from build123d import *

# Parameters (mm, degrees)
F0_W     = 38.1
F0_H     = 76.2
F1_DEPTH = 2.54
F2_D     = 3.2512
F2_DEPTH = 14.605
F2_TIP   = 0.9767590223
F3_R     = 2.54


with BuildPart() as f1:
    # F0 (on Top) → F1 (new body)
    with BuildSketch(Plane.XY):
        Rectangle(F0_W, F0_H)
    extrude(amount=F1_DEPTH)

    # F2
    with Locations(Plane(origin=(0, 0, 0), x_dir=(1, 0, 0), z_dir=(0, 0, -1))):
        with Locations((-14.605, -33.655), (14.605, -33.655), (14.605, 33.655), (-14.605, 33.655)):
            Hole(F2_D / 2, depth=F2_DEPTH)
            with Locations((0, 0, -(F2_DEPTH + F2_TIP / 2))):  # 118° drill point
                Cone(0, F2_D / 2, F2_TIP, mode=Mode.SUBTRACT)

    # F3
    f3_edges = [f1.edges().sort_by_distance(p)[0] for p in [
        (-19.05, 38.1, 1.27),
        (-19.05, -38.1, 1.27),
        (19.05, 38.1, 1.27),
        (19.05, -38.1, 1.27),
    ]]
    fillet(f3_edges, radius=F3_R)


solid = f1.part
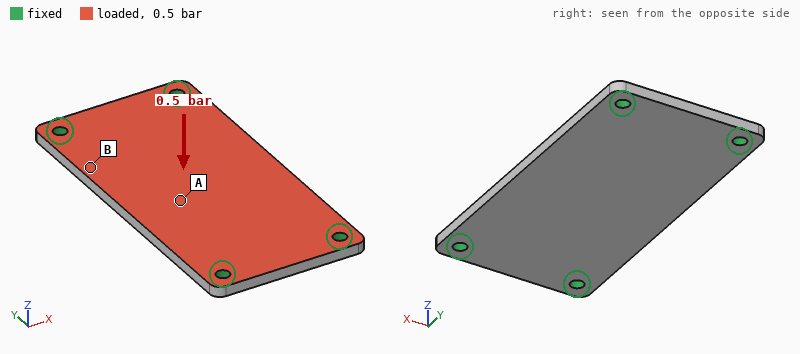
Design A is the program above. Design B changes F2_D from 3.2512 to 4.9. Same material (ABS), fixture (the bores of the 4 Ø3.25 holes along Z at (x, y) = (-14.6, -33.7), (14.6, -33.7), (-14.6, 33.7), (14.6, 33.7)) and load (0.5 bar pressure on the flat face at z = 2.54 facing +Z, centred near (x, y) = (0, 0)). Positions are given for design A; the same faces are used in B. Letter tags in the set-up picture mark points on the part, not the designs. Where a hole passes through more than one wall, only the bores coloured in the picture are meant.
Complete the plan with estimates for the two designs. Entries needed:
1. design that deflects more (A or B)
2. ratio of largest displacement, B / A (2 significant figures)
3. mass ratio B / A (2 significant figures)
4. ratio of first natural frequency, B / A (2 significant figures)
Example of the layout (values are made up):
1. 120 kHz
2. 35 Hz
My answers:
1. A
2. 0.86
3. 0.99
4. 1.1
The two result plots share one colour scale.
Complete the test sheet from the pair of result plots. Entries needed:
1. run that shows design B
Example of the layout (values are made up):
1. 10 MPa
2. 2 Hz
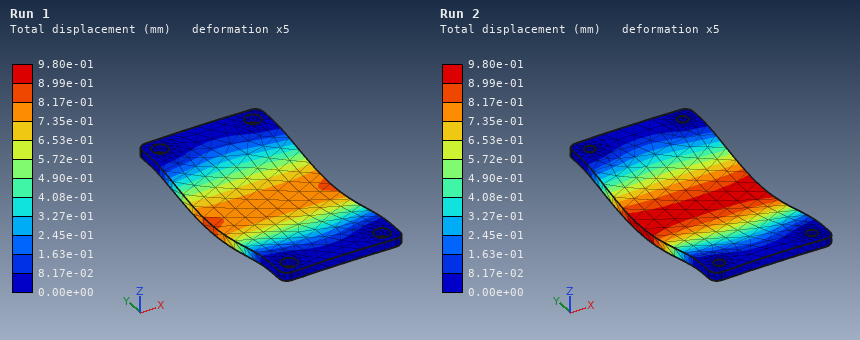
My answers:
1. Run 1
